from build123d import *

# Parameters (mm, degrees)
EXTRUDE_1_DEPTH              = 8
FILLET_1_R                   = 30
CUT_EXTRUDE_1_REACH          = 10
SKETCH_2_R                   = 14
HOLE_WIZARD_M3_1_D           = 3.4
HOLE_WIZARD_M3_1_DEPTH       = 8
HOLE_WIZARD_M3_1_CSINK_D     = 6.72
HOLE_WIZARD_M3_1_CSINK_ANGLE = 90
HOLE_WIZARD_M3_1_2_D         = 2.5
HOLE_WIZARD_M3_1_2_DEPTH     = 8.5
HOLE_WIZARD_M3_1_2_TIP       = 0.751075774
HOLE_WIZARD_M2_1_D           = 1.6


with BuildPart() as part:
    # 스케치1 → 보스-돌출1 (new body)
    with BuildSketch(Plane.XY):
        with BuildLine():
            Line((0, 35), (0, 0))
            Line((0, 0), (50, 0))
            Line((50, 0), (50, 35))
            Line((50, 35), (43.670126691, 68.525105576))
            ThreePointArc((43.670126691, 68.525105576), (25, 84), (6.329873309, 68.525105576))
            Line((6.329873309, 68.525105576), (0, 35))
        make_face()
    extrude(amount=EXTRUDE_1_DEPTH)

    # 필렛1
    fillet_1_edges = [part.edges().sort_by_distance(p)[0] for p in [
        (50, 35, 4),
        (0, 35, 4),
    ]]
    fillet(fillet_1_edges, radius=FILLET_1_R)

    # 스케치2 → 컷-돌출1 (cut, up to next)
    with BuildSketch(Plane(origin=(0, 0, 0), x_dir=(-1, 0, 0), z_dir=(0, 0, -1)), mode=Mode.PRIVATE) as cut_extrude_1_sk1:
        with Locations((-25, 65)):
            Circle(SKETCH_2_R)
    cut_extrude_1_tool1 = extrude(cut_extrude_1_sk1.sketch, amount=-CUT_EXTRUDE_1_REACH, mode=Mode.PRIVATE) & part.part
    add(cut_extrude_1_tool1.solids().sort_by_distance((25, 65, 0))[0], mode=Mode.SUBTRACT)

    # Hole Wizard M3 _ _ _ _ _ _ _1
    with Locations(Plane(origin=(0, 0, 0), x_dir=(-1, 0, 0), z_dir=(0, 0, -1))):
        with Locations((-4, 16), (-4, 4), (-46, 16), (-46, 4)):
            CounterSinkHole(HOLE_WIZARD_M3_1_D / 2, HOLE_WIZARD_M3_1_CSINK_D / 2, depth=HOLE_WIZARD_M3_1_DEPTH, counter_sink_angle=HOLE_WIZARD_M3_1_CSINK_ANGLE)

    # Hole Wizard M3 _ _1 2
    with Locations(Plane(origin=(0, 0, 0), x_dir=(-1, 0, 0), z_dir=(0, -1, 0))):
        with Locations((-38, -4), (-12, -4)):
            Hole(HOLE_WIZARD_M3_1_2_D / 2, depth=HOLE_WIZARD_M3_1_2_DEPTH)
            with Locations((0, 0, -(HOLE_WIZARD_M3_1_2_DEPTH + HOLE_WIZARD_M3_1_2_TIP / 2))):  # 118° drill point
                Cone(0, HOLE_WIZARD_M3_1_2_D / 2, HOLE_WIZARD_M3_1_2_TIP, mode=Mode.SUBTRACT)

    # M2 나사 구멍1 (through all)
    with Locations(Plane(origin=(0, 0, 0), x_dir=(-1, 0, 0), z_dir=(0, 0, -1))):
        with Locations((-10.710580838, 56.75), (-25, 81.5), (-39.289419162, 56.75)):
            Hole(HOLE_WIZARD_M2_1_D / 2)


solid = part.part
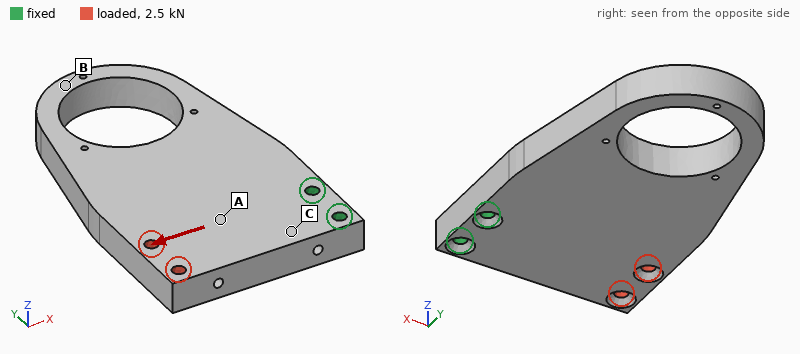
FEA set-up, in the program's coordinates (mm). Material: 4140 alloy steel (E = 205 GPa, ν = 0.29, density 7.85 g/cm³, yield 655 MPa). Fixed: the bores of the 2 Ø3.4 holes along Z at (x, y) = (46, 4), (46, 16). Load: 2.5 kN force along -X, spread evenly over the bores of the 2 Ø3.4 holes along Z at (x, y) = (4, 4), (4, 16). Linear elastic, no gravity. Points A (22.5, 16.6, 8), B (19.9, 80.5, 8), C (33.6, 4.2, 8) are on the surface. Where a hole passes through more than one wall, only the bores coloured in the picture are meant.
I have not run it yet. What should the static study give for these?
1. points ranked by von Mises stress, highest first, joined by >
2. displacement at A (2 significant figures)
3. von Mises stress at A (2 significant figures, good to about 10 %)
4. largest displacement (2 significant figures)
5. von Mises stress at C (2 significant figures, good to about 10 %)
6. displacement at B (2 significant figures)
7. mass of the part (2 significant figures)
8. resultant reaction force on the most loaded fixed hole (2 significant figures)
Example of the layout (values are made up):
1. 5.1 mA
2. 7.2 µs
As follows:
1. C > A > B
2. 2.8 µm
3. 15 MPa
4. 9.3 µm
5. 25 MPa
6. 2.3 µm
7. 190 g
8. 1.3 kN
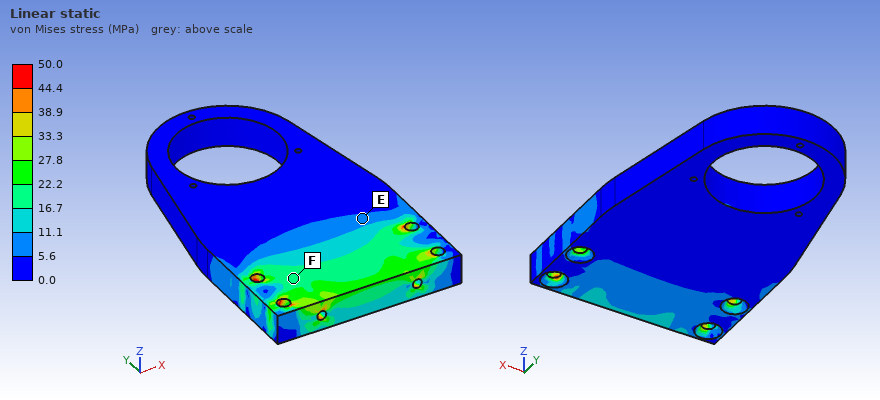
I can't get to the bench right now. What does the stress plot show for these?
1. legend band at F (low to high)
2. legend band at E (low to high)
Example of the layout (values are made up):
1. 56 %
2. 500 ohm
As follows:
1. 16.7 to 22.2 MPa
2. 5.6 to 11.1 MPa
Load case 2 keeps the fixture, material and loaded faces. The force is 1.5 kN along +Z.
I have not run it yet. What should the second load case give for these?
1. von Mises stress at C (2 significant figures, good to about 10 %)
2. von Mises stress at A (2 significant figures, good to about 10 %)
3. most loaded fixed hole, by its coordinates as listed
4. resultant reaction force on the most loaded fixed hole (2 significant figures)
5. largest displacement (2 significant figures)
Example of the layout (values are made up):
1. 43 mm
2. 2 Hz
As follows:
1. 140 MPa
2. 65 MPa
3. (46, 16)
4. 860 N
5. 0.20 mm
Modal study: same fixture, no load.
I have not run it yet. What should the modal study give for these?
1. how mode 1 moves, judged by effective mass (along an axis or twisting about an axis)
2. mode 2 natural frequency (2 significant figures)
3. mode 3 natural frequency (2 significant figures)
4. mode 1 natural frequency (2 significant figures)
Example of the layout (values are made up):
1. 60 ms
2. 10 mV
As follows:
1. along Z
2. 2600 Hz
3. 3000 Hz
4. 1400 Hz
